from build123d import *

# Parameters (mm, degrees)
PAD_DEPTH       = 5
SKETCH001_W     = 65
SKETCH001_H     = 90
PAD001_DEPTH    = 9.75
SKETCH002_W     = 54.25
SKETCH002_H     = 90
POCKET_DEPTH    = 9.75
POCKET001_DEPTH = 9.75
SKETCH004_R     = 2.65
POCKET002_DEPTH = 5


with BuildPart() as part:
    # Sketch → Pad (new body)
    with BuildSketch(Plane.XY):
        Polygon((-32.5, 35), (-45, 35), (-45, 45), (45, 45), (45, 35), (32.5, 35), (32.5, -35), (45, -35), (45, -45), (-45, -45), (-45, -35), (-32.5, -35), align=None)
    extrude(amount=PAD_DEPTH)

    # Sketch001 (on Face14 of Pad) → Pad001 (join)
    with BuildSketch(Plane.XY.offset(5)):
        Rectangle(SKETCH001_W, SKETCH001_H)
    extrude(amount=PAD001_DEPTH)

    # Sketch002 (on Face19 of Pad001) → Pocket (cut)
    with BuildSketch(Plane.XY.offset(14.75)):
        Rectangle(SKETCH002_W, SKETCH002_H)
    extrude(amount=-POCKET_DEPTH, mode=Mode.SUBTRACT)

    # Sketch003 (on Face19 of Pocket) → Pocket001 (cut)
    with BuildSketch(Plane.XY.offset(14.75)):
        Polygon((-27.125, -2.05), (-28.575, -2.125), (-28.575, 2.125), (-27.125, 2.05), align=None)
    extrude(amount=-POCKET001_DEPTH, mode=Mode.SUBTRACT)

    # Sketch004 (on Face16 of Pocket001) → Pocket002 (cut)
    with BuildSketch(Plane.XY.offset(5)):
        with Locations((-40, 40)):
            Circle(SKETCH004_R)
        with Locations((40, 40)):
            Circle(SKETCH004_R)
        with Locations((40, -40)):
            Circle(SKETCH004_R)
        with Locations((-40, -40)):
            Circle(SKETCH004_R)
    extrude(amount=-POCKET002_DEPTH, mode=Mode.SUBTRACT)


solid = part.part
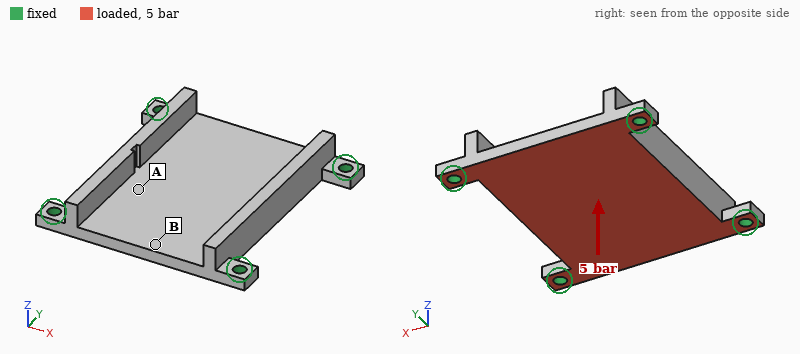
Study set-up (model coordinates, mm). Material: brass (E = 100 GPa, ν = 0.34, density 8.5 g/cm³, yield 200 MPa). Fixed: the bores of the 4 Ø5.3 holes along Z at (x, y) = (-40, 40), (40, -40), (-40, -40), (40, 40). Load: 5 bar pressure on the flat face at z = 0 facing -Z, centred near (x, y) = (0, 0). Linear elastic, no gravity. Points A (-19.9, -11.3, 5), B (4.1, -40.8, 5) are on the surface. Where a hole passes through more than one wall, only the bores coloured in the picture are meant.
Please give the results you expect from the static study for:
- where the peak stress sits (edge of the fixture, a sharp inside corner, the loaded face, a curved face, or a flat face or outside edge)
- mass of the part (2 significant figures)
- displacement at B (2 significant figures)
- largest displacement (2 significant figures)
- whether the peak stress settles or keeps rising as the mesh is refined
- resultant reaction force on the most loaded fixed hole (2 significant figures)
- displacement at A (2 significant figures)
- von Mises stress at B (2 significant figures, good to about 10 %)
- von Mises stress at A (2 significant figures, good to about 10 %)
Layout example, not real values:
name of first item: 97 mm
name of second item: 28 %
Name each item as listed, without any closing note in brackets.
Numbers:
where the peak stress sits: edge of the fixture
mass of the part: 350 g
displacement at B: 0.086 mm
largest displacement: 0.10 mm
whether the peak stress settles or keeps rising as the mesh is refined: keeps rising
resultant reaction force on the most loaded fixed hole: 810 N
displacement at A: 0.074 mm
von Mises stress at B: 48 MPa
von Mises stress at A: 22 MPa
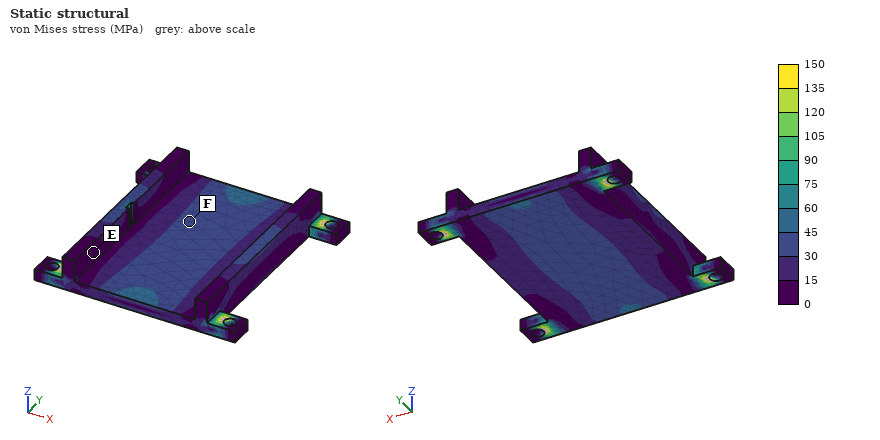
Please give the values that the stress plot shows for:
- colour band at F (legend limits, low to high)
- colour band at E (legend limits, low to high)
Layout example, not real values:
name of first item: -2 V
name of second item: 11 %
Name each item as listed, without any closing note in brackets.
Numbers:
colour band at F: 30 to 45 MPa
colour band at E: 0 to 15 MPa
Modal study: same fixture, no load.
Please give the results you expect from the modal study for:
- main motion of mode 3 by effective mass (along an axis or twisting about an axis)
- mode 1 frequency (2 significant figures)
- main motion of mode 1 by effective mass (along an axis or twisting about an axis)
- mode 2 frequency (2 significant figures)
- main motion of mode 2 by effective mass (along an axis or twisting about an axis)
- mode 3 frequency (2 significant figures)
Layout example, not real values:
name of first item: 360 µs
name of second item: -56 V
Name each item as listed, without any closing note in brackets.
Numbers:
main motion of mode 3 by effective mass: twisting about Y
mode 1 frequency: 1800 Hz
main motion of mode 1 by effective mass: along Z
mode 2 frequency: 3000 Hz
main motion of mode 2 by effective mass: twisting about X
mode 3 frequency: 3700 Hz
